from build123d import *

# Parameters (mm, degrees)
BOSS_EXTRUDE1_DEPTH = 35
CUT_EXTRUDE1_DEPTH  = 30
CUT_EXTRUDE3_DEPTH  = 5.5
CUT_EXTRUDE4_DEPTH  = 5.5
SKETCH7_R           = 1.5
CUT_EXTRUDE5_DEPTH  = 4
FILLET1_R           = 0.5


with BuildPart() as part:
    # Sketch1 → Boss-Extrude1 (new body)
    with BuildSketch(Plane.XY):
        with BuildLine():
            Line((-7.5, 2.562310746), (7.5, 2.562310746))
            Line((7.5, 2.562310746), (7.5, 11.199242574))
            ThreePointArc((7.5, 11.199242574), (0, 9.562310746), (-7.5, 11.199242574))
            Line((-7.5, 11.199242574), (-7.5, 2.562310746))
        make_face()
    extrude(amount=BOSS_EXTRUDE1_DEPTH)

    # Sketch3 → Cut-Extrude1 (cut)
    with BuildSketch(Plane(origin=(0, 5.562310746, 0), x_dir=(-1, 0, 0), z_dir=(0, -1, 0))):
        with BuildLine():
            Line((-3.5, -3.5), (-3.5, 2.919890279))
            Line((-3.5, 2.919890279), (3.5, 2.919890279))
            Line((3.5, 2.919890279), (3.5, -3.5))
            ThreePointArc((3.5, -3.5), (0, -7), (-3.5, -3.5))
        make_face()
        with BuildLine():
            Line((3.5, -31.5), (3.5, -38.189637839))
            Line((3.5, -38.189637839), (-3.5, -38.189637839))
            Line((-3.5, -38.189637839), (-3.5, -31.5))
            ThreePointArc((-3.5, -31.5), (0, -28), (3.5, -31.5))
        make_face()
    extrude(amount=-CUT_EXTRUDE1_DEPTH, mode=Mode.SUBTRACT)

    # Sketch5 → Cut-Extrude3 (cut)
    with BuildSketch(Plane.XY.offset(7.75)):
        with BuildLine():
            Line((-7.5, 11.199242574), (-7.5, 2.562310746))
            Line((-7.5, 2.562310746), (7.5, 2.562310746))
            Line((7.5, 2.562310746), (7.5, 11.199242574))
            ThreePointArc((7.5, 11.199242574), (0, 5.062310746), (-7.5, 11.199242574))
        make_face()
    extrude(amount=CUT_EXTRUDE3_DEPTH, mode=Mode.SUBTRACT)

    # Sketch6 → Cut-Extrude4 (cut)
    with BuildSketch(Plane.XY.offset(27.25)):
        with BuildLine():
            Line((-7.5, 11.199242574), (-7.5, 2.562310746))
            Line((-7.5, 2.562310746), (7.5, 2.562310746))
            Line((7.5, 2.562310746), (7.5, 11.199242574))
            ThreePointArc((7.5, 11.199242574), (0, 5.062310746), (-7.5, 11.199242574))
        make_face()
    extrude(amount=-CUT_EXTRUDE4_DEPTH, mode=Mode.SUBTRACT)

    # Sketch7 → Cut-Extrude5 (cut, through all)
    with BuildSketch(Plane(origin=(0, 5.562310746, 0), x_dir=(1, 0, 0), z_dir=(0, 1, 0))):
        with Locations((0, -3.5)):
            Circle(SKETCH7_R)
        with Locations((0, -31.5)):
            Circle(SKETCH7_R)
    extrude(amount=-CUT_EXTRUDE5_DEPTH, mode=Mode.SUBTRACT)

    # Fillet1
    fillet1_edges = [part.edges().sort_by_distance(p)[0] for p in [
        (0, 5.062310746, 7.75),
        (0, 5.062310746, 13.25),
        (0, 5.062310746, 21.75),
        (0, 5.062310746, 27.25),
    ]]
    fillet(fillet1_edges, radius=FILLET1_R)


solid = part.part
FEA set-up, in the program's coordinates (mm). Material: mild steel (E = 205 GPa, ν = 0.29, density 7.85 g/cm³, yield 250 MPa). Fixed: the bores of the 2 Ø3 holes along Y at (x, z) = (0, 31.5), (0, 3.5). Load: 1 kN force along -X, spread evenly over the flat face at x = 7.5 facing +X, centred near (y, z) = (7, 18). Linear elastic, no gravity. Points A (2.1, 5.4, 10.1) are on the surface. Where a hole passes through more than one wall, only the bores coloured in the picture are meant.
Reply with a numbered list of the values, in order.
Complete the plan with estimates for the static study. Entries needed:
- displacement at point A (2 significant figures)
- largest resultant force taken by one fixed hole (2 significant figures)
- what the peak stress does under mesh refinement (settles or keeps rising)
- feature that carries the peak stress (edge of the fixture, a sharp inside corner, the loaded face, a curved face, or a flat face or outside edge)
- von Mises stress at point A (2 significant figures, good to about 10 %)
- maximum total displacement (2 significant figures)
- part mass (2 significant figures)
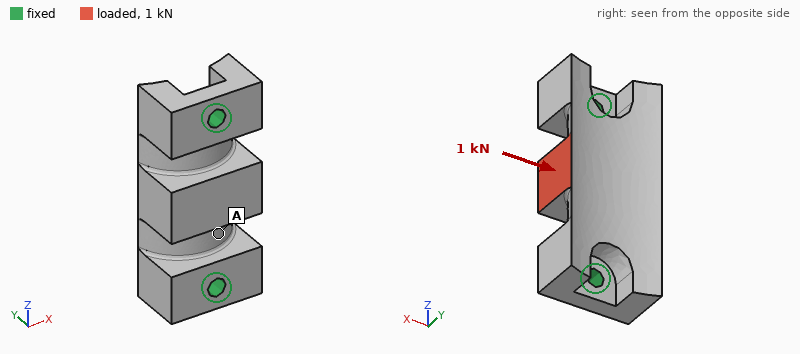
1. 3.1 µm
2. 500 N
3. keeps rising
4. edge of the fixture
5. 22 MPa
6. 8.0 µm
7. 23 g
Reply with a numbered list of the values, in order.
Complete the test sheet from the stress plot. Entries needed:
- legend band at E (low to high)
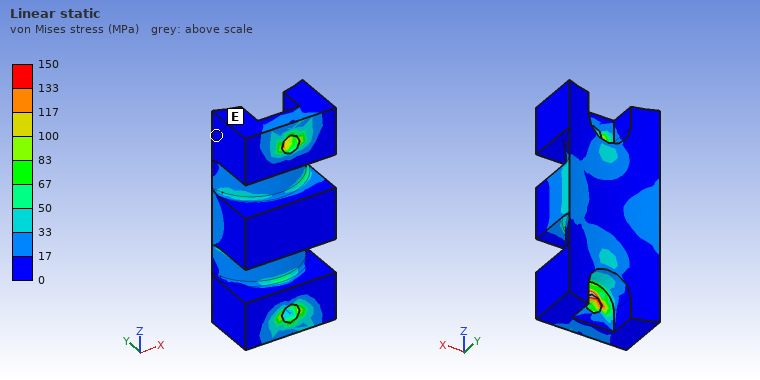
1. 0 to 17 MPa
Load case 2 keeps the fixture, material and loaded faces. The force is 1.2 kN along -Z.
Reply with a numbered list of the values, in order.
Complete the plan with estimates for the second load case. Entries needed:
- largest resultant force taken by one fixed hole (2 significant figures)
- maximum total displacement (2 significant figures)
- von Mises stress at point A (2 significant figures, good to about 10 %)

1. 690 N
2. 7.4 µm
3. 58 MPa
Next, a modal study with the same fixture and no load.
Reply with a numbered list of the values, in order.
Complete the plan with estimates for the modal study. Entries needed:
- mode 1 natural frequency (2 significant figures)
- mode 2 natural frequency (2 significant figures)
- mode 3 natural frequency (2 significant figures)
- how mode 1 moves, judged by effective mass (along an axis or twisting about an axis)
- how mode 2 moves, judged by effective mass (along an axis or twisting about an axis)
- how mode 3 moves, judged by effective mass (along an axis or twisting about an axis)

1. 15 kHz
2. 22 kHz
3. 25 kHz
4. along X
5. along Y
6. along X
